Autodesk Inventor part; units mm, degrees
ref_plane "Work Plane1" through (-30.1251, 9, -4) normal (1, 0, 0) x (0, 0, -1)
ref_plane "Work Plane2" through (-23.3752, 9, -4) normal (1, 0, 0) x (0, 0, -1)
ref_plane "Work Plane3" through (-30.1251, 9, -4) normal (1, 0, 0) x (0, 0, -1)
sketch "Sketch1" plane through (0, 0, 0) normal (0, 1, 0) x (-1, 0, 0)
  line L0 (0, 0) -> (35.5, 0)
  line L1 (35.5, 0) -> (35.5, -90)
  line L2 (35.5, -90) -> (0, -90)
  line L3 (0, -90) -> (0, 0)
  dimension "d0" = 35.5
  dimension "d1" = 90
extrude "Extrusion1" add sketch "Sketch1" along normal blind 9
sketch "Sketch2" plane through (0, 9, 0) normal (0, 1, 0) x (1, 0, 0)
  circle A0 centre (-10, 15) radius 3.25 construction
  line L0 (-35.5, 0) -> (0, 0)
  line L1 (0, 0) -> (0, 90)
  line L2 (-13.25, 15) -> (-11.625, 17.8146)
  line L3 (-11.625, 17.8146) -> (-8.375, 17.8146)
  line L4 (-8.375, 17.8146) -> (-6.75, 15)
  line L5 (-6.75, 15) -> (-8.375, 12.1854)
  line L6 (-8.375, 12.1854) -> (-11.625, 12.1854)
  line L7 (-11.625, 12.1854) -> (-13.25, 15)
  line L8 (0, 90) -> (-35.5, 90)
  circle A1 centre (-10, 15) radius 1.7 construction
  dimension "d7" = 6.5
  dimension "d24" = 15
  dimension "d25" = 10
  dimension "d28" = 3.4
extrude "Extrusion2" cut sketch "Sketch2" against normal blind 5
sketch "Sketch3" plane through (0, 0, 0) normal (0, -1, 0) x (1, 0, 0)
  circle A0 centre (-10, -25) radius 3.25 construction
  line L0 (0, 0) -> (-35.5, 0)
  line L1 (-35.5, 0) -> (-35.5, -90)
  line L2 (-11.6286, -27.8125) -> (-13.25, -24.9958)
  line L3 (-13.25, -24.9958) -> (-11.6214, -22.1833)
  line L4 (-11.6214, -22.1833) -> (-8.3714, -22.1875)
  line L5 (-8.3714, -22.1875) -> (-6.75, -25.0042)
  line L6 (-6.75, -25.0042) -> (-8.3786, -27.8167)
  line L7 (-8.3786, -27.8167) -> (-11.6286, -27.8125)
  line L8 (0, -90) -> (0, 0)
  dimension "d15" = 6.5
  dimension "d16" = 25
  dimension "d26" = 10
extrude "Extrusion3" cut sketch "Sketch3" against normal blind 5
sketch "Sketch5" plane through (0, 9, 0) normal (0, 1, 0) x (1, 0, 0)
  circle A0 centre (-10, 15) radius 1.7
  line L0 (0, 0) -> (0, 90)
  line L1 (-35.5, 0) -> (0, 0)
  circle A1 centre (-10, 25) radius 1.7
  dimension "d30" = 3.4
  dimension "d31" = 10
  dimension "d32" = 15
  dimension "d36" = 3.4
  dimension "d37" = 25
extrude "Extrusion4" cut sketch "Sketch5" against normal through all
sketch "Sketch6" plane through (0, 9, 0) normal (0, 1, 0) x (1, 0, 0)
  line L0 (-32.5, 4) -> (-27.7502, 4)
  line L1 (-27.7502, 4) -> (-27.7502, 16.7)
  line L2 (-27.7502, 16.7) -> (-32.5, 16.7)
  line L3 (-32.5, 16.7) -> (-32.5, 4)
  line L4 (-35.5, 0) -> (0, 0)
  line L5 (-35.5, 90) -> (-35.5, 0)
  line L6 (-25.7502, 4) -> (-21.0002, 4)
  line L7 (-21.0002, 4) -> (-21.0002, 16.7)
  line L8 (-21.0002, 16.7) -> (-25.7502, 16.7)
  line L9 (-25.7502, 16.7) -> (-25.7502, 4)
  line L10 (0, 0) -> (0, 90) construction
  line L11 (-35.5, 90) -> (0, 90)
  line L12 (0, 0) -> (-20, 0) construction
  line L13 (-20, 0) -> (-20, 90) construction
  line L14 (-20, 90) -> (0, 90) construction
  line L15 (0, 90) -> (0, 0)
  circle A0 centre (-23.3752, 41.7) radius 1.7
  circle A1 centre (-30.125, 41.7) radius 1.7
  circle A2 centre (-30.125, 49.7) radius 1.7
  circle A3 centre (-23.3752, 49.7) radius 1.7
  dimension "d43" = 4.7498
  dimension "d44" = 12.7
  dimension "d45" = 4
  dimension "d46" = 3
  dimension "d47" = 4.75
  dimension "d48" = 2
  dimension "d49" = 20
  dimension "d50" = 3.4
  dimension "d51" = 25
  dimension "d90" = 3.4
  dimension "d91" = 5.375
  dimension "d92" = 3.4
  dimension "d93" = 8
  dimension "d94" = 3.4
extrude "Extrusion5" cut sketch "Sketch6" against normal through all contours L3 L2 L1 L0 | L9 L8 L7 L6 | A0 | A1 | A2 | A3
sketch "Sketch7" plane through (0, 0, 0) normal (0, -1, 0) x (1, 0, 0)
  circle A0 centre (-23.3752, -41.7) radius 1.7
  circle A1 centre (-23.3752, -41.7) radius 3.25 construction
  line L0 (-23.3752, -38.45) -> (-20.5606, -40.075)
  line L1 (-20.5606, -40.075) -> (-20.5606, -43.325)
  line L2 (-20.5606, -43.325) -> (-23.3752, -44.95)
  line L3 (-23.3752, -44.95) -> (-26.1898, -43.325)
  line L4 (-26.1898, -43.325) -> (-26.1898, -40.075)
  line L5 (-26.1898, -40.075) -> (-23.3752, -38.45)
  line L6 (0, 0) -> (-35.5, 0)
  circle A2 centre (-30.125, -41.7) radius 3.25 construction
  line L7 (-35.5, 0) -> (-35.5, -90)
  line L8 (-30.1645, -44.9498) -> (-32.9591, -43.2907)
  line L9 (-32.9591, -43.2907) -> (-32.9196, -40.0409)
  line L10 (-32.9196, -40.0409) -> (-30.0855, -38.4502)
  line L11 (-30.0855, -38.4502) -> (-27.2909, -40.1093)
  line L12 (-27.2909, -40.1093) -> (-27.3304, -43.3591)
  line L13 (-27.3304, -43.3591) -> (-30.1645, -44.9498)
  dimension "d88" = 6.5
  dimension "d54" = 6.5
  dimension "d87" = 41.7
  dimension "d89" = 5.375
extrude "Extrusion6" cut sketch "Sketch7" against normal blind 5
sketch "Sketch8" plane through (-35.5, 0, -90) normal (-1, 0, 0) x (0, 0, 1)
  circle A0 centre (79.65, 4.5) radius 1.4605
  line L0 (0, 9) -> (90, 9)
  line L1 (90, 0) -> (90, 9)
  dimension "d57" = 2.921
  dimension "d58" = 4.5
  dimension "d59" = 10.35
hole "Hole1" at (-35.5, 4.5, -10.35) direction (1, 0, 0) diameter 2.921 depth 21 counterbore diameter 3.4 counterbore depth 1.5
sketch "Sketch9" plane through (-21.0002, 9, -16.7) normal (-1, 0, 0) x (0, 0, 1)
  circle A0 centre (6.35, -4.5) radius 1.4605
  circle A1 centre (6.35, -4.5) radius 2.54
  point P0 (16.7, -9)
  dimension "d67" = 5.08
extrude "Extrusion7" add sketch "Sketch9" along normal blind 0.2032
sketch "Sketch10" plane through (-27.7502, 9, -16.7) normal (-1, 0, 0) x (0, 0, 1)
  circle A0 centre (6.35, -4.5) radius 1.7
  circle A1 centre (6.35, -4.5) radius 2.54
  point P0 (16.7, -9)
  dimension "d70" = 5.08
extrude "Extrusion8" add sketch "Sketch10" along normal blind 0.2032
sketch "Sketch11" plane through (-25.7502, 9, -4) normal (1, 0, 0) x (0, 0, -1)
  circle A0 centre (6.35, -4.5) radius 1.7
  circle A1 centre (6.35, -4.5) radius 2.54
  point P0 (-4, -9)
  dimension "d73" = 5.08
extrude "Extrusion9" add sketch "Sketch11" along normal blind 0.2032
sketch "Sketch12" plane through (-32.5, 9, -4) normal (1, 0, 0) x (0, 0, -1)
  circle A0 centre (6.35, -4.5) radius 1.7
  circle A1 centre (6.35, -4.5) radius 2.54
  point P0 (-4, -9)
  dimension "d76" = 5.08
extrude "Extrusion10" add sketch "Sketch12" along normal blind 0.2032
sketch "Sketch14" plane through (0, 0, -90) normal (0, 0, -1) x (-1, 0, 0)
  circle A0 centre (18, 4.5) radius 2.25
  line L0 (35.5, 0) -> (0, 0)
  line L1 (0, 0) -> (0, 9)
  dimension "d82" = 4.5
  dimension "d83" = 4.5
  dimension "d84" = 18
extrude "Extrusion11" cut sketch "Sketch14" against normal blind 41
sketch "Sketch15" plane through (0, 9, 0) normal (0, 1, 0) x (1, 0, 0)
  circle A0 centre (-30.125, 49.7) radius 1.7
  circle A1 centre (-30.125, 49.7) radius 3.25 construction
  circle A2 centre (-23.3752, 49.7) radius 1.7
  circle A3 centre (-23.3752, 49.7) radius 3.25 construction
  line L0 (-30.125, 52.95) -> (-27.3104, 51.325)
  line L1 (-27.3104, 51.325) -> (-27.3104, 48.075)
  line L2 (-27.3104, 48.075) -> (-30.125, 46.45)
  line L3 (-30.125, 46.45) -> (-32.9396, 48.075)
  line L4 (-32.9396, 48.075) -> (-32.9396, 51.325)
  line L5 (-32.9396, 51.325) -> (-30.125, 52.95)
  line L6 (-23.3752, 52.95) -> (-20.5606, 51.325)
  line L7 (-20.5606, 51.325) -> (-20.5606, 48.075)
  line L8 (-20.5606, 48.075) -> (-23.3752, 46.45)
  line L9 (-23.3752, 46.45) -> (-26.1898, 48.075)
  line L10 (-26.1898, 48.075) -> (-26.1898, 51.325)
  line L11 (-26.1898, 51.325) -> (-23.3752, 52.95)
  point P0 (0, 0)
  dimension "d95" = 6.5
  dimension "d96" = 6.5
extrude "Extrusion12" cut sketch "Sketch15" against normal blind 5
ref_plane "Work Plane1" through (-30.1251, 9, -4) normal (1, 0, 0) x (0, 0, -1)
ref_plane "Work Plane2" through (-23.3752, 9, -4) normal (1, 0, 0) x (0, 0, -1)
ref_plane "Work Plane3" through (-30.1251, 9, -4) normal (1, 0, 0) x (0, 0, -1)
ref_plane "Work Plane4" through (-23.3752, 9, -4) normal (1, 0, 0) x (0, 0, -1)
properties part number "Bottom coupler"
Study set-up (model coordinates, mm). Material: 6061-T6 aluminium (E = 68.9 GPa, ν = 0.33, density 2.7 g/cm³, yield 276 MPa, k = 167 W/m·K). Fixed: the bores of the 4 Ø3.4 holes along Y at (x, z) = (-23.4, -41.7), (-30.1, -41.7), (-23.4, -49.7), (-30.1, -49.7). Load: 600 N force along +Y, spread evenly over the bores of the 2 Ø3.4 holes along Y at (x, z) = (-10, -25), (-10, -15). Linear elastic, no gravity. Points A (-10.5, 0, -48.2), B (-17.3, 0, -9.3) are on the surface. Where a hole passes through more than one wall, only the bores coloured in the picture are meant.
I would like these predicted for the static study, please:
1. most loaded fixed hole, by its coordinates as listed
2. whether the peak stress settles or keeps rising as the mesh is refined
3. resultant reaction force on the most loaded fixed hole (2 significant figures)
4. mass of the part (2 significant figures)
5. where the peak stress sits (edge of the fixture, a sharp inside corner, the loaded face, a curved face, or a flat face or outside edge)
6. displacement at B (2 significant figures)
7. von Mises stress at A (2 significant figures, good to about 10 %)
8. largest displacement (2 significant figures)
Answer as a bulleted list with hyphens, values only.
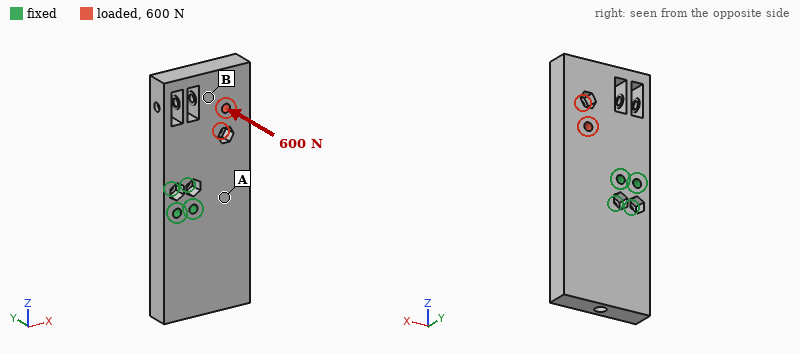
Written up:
- (-23.4, -41.7)
- keeps rising
- 1.5 kN
- 70 g
- edge of the fixture
- 0.064 mm
- 19 MPa
- 0.10 mm
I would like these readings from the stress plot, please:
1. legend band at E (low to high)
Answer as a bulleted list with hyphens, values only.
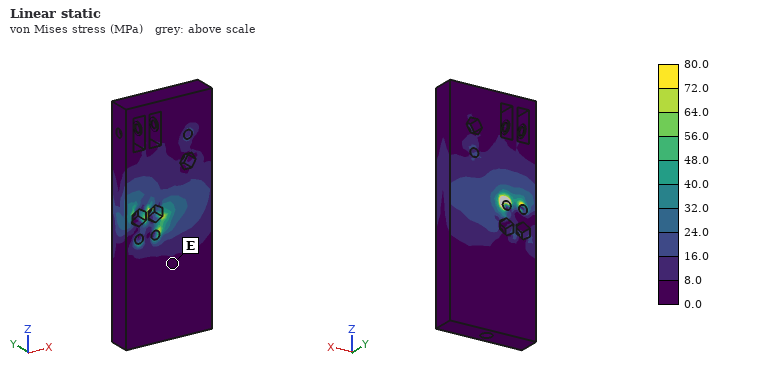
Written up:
- 0.0 to 8.0 MPa
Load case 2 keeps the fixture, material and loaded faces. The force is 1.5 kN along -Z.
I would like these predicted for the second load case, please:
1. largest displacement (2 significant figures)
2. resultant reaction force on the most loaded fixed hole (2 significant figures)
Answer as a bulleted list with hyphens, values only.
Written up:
- 32 µm
- 1.5 kN
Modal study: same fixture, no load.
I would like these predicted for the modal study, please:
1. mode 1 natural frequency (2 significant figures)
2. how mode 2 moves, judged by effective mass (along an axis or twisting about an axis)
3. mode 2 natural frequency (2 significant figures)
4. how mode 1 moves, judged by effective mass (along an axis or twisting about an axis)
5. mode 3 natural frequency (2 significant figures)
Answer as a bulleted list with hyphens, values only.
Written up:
- 2800 Hz
- along Y
- 3500 Hz
- twisting about X
- 4500 Hz
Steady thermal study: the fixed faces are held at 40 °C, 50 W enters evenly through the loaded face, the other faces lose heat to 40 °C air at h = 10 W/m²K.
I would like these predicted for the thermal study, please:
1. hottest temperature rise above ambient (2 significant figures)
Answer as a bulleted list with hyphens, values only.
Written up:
- 41 K
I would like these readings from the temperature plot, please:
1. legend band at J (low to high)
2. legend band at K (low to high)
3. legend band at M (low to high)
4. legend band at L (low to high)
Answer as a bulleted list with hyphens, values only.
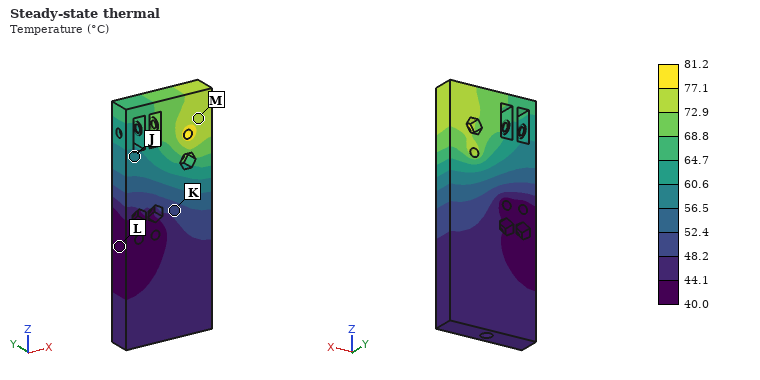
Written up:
- 56.5 to 60.6 °C
- 48.2 to 52.4 °C
- 72.9 to 77.1 °C
- 40.0 to 44.1 °C
